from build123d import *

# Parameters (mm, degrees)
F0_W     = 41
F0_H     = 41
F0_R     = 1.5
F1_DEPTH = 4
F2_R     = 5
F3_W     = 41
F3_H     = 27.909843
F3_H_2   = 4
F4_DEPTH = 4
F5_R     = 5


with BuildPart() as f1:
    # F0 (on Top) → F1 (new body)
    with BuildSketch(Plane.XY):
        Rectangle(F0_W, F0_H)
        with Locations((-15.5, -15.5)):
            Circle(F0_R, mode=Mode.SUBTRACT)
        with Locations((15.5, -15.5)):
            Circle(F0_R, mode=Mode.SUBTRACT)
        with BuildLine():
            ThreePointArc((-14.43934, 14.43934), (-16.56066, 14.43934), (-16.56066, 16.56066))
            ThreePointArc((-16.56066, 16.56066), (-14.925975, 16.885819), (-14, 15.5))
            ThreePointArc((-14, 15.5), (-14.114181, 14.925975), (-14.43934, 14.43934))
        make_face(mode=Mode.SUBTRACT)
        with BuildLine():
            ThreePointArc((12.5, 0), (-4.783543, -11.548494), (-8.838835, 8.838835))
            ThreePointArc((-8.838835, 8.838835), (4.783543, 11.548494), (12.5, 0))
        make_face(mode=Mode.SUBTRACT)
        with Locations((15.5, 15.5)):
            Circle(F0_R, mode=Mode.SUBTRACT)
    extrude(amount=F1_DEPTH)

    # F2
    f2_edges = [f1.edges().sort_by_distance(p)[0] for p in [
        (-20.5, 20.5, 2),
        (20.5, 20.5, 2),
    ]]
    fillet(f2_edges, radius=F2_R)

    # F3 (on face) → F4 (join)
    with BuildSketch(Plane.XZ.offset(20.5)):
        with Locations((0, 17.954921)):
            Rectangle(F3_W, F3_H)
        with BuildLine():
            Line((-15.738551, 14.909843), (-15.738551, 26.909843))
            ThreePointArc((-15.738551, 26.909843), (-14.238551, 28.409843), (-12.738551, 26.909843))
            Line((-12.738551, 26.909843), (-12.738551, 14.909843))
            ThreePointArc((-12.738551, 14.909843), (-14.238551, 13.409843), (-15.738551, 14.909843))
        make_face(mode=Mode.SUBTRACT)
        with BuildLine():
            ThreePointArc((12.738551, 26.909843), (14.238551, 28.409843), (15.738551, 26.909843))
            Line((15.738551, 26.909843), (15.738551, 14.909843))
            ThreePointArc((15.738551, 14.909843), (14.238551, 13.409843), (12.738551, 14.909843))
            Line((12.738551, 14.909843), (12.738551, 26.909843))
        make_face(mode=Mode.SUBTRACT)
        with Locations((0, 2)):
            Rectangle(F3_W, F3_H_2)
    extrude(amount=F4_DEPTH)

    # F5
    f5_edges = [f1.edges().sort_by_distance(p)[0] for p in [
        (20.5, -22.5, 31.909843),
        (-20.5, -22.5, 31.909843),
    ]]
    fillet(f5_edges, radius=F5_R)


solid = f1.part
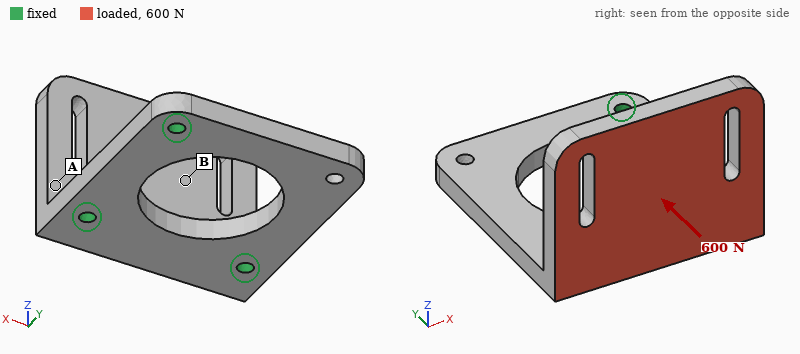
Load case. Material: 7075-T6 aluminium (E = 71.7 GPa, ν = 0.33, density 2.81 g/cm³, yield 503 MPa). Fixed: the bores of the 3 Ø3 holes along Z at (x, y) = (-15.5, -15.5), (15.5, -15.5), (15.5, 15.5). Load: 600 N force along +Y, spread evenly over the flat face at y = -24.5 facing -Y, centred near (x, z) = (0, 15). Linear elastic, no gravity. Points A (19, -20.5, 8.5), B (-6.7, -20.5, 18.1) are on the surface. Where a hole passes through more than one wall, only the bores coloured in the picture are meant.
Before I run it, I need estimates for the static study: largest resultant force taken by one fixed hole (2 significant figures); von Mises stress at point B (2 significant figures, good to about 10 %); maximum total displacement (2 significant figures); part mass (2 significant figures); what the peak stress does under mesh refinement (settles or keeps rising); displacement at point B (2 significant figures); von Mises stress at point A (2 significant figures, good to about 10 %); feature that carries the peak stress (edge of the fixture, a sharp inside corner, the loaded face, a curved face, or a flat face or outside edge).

320 N
19 MPa
0.23 mm
27 g
keeps rising
0.11 mm
40 MPa
edge of the fixture
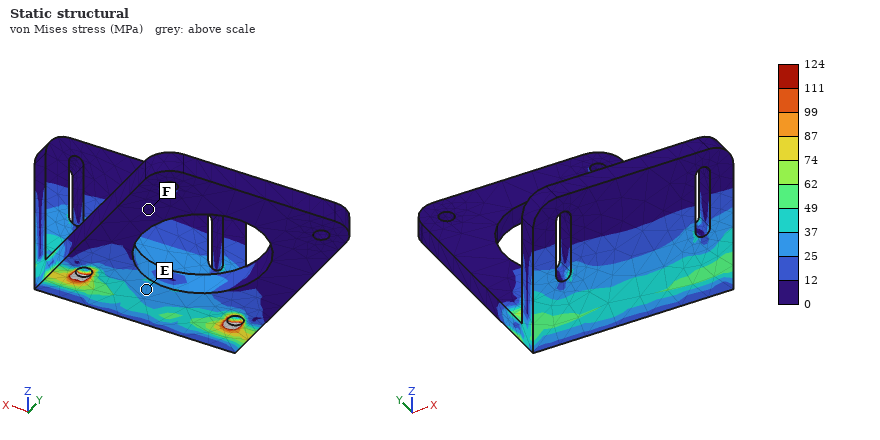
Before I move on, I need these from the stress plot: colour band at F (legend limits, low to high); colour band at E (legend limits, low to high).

0 to 12 MPa
25 to 37 MPa
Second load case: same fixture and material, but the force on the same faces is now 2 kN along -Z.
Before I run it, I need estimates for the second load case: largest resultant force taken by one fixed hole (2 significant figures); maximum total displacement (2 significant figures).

1.0 kN
0.27 mm
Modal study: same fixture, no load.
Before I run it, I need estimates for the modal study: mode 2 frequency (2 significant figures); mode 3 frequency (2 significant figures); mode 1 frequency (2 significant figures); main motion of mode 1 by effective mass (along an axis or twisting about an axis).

4400 Hz
6200 Hz
2700 Hz
along Y
